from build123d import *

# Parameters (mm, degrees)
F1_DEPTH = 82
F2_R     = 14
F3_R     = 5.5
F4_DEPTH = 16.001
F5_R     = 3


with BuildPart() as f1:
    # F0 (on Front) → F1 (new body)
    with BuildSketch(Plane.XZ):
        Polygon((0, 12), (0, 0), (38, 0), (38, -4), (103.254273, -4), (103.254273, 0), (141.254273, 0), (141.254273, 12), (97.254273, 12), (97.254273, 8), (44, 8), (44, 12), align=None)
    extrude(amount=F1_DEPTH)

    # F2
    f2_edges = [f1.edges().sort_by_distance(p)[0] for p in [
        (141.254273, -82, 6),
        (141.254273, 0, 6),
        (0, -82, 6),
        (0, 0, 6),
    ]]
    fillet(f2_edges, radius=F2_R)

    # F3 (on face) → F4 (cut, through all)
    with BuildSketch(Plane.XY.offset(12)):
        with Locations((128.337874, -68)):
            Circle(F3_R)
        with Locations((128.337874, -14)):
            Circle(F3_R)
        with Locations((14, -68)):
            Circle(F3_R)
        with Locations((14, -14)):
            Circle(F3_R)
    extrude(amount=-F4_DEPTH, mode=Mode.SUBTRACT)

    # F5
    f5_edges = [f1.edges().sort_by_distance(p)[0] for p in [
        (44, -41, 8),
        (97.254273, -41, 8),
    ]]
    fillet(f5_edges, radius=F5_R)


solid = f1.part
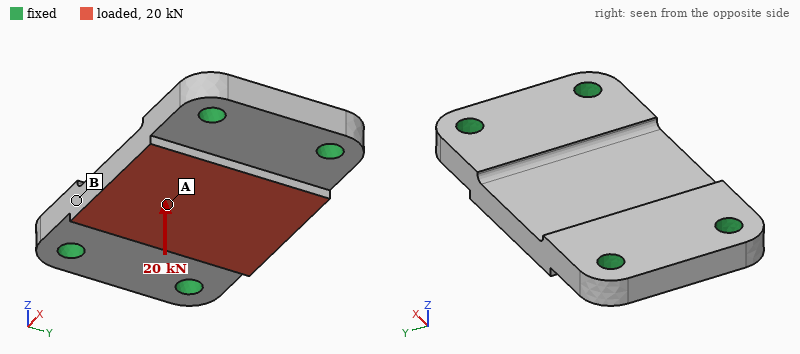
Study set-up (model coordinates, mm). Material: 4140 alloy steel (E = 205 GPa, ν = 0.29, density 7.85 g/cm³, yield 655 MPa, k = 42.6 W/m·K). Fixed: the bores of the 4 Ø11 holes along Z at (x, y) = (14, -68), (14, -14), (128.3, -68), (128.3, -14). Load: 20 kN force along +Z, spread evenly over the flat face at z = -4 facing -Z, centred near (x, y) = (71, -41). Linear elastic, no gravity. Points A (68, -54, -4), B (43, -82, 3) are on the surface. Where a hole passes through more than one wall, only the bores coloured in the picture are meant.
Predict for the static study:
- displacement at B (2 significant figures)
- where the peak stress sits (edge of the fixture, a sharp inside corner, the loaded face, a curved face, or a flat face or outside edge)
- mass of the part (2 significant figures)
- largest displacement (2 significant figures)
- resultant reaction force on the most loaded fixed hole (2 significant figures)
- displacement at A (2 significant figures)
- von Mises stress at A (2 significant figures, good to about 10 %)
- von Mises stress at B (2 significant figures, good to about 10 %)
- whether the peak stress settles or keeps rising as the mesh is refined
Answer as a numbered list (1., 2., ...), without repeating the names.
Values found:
1. 25 µm
2. edge of the fixture
3. 1.1 kg
4. 45 µm
5. 8.3 kN
6. 43 µm
7. 66 MPa
8. 28 MPa
9. keeps rising
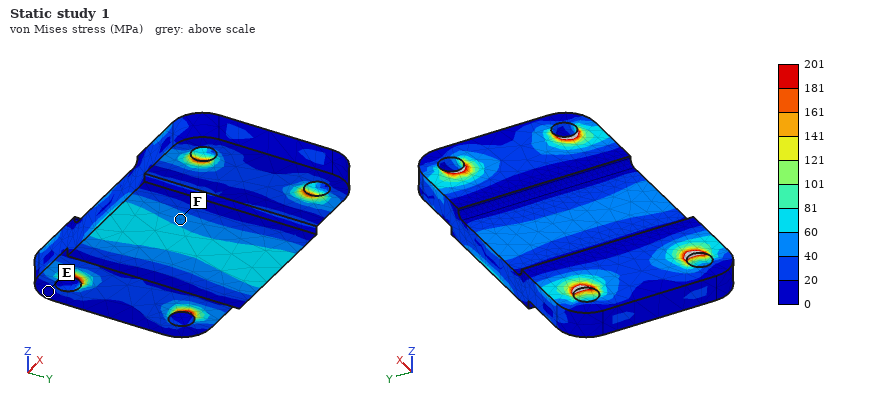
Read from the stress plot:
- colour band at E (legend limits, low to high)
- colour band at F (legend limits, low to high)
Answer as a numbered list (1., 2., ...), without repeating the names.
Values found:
1. 0 to 20 MPa
2. 40 to 60 MPa
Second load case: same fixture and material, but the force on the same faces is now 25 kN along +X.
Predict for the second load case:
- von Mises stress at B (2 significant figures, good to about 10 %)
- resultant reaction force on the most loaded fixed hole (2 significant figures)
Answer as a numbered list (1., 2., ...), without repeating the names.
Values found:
1. 16 MPa
2. 6.5 kN
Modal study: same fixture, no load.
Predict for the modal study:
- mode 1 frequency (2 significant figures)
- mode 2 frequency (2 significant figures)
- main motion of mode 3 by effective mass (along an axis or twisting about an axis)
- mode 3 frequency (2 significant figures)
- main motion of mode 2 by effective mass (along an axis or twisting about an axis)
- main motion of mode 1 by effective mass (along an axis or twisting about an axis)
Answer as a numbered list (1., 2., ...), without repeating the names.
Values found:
1. 4900 Hz
2. 6600 Hz
3. twisting about Y
4. 11 kHz
5. twisting about X
6. along Z
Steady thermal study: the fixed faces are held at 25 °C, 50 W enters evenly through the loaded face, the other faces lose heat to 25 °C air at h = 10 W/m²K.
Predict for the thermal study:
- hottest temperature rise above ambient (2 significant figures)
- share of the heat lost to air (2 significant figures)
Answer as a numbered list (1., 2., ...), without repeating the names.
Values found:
1. 25 K
2. 4.9 %
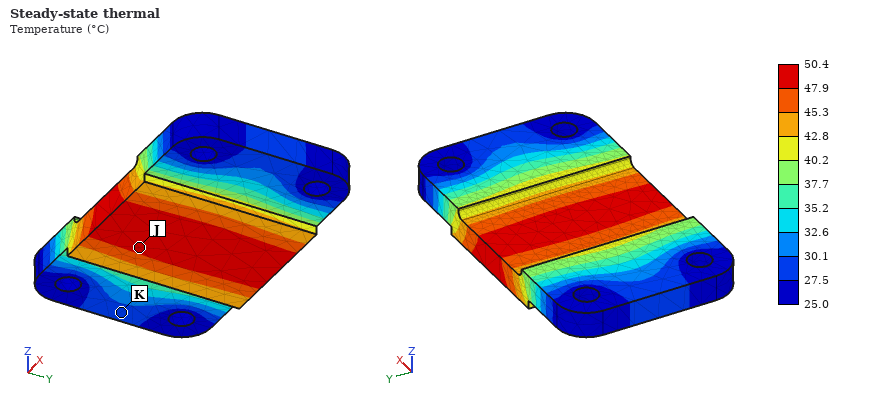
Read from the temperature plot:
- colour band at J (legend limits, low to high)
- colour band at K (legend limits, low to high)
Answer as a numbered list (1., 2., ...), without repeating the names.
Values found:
1. 47.9 to 50.4 °C
2. 27.5 to 30.1 °C
